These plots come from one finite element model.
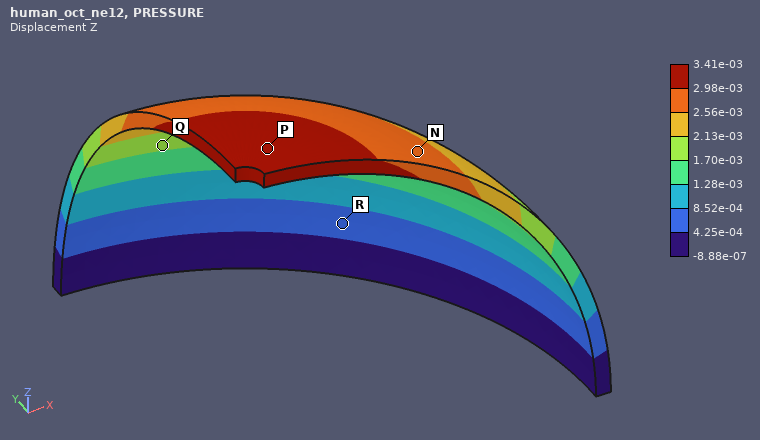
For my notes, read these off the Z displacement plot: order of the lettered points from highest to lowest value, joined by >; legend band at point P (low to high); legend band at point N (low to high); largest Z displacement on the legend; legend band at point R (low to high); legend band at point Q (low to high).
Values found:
P > N > Q > R
2.98e-03 to 3.41e-03
2.56e-03 to 2.98e-03
3.41e-03
4.25e-04 to 8.52e-04
1.70e-03 to 2.13e-03
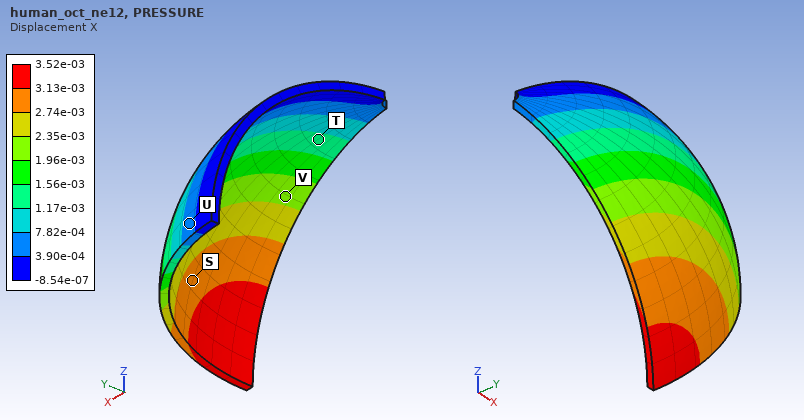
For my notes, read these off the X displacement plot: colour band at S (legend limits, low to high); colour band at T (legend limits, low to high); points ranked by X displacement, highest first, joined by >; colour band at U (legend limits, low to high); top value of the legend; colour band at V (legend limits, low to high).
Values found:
2.74e-03 to 3.13e-03
1.17e-03 to 1.56e-03
S > V > T > U
3.90e-04 to 7.82e-04
3.52e-03
1.96e-03 to 2.35e-03
